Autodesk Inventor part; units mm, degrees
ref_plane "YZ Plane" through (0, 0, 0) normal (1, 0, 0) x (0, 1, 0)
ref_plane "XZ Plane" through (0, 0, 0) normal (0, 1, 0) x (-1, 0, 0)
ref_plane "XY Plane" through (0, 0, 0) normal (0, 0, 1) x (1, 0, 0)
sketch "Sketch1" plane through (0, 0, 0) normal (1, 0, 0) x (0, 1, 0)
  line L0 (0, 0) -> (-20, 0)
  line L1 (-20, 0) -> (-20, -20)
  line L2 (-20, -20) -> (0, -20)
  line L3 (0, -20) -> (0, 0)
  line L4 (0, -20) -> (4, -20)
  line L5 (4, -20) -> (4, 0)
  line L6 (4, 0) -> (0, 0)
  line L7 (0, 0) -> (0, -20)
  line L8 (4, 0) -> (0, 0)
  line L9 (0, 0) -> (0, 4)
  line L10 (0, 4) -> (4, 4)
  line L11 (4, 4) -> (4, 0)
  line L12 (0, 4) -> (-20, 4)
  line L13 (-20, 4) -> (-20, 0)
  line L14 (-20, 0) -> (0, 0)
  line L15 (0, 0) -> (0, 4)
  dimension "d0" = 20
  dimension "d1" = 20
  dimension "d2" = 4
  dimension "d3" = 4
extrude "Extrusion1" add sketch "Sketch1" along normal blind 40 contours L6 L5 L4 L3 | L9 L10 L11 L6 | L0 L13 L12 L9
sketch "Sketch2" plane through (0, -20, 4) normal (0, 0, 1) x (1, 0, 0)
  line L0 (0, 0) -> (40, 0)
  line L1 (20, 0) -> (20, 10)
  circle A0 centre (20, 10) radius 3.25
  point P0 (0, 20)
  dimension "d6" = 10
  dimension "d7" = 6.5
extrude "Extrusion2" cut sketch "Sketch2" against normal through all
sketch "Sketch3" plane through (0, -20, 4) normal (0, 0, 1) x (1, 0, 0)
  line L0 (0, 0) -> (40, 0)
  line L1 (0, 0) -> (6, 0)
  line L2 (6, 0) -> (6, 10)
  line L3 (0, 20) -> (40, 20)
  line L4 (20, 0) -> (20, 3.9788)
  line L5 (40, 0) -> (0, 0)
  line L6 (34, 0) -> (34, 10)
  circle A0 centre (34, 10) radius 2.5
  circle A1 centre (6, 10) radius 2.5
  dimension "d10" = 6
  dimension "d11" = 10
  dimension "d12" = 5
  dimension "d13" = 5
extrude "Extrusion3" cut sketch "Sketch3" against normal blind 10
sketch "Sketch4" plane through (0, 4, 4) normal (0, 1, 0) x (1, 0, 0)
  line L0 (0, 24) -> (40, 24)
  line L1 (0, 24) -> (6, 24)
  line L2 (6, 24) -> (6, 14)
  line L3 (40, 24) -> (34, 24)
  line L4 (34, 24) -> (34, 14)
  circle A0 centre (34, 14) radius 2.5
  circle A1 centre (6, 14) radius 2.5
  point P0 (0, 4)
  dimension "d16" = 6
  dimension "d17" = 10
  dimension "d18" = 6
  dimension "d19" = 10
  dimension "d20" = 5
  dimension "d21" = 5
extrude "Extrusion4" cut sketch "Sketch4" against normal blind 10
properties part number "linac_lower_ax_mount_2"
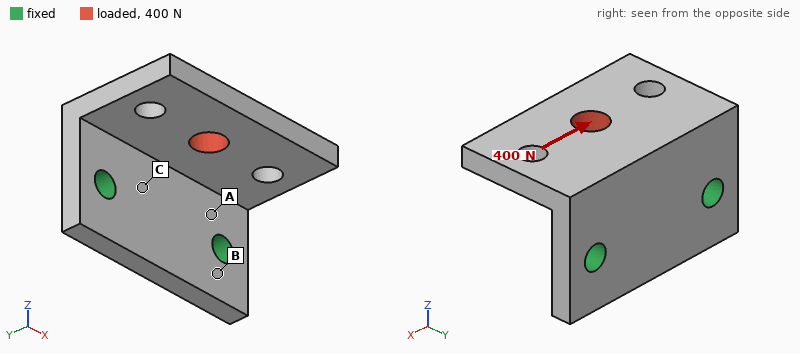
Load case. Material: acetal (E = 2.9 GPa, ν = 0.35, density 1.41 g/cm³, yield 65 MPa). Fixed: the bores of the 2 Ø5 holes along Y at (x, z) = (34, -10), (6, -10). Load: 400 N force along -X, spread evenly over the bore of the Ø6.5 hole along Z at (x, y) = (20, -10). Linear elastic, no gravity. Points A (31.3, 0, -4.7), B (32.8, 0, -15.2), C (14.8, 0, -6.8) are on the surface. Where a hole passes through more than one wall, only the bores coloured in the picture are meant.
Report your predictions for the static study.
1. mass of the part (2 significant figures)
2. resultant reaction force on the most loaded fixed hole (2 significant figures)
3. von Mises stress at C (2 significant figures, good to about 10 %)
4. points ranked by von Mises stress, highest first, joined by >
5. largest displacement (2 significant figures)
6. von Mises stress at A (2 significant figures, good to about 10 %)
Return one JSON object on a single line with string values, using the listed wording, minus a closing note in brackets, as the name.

{"mass of the part": "9.3 g", "resultant reaction force on the most loaded fixed hole": "300 N", "von Mises stress at C": "10 MPa", "points ranked by von Mises stress, highest first, joined by >": "A > C > B", "largest displacement": "0.50 mm", "von Mises stress at A": "16 MPa"}
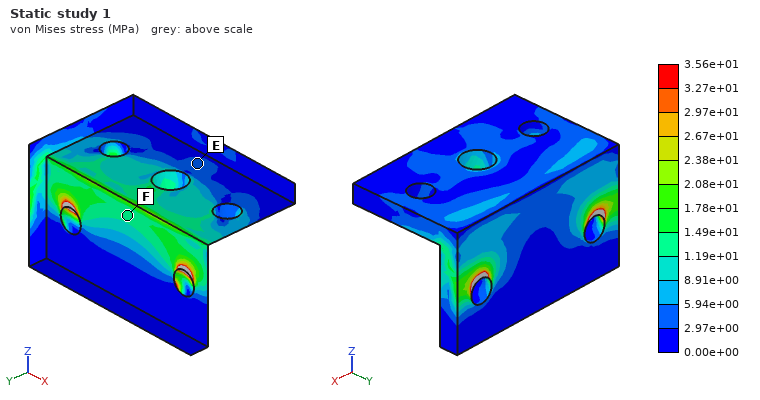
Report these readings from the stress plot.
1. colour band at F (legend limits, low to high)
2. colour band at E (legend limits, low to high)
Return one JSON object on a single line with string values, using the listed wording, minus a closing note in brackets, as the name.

{"colour band at F": "1.19e+01 to 1.49e+01 MPa", "colour band at E": "2.97e+00 to 5.94e+00 MPa"}
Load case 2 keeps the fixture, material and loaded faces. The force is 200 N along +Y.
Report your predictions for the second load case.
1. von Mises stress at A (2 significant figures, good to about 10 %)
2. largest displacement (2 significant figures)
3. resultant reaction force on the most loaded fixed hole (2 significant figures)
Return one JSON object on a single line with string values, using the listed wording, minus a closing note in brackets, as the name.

{"von Mises stress at A": "14 MPa", "largest displacement": "0.52 mm", "resultant reaction force on the most loaded fixed hole": "100 N"}
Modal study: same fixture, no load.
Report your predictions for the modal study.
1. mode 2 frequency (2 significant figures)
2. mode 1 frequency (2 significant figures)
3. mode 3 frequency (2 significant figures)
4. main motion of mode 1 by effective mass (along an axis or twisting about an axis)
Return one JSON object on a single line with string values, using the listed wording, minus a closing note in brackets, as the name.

{"mode 2 frequency": "2000 Hz", "mode 1 frequency": "1100 Hz", "mode 3 frequency": "3100 Hz", "main motion of mode 1 by effective mass": "along Z"}
